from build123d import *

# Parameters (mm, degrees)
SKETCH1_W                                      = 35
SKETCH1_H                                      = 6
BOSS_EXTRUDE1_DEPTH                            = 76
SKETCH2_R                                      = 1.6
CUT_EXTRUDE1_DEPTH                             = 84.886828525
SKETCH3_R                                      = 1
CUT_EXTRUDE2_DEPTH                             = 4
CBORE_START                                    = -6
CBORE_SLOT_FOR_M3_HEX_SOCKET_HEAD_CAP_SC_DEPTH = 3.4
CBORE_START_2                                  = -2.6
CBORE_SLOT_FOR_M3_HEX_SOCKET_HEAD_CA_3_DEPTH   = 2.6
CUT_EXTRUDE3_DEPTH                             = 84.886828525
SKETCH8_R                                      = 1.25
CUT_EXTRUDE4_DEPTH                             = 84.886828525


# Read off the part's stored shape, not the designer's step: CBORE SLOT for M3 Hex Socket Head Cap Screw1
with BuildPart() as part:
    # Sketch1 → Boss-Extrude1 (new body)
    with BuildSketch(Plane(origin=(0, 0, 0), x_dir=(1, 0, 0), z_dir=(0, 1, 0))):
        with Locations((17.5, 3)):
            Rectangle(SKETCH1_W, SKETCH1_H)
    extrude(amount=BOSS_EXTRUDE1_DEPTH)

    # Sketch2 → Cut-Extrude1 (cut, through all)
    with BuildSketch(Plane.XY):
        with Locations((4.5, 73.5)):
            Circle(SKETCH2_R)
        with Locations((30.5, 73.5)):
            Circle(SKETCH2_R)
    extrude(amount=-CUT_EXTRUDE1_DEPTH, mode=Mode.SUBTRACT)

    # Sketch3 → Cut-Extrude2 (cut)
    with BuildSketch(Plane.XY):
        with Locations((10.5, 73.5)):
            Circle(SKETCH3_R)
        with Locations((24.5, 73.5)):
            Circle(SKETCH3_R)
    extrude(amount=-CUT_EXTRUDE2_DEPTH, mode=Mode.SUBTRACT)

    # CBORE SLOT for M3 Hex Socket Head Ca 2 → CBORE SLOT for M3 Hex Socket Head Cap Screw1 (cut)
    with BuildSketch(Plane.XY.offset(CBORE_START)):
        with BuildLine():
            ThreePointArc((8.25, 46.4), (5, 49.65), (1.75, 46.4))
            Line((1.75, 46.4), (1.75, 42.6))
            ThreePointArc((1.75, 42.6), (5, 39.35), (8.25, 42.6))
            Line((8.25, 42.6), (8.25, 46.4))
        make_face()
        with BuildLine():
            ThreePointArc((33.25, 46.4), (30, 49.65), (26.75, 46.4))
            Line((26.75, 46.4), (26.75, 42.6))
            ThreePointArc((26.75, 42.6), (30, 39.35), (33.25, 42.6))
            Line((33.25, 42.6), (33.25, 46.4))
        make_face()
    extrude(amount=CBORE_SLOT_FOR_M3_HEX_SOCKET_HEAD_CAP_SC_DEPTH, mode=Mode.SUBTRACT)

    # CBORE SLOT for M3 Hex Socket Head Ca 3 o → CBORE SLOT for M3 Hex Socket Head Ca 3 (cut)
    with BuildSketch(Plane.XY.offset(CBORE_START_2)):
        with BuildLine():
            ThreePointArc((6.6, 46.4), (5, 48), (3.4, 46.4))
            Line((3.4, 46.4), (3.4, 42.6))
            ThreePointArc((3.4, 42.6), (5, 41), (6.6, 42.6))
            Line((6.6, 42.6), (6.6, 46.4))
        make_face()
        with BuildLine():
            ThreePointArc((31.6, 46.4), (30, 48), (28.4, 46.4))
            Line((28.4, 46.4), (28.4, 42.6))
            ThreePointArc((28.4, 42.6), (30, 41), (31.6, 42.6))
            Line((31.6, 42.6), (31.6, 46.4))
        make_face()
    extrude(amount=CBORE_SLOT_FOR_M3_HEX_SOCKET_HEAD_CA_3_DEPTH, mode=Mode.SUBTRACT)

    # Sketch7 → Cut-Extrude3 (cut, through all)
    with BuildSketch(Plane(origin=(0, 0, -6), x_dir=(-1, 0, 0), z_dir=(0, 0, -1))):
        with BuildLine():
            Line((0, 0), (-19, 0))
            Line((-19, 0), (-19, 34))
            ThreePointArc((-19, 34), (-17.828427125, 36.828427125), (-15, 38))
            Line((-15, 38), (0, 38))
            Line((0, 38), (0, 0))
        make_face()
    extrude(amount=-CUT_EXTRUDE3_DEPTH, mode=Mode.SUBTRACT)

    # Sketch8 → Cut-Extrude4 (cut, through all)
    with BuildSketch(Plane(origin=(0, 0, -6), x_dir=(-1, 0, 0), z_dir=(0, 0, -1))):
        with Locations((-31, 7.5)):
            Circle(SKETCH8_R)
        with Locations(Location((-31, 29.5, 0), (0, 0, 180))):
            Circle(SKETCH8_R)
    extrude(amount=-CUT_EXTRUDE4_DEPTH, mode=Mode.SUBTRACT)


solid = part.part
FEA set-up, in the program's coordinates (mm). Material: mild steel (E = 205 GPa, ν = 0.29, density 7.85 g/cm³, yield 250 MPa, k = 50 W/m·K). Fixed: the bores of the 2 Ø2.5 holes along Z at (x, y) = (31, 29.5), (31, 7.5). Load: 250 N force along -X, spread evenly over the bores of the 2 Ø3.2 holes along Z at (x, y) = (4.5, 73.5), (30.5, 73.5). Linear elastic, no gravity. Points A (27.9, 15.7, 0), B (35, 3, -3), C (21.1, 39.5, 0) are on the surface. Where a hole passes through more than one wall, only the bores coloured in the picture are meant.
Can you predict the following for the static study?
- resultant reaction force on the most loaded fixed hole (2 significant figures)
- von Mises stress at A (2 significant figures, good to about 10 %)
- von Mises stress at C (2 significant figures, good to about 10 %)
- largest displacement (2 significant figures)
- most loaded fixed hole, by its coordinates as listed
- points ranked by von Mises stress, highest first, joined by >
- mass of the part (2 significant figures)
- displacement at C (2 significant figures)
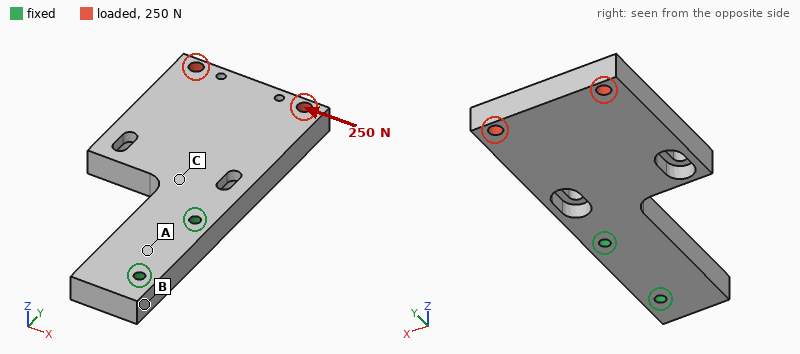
800 N
12 MPa
20 MPa
31 µm
(31, 29.5)
C > A > B
86 g
4.8 µm
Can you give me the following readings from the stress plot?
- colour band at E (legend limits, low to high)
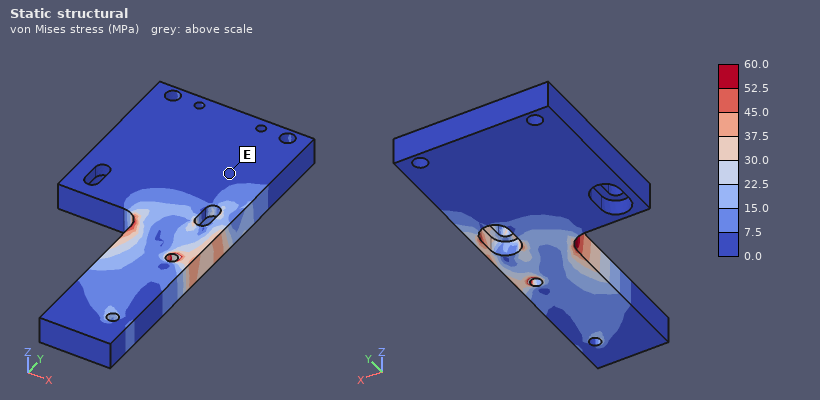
0.0 to 7.5 MPa
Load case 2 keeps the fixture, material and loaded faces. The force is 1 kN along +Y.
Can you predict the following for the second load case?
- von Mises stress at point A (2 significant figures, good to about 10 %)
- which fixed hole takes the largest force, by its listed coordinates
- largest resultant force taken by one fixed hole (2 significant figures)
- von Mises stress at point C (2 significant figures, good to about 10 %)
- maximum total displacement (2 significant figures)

16 MPa
(31, 7.5)
820 N
26 MPa
31 µm
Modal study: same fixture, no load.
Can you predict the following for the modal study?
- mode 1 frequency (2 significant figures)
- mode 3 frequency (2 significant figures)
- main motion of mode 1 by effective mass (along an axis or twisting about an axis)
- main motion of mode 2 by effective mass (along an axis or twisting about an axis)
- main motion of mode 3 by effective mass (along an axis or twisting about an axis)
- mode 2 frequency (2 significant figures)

1300 Hz
3600 Hz
along Z
along X
twisting about Y
2900 Hz
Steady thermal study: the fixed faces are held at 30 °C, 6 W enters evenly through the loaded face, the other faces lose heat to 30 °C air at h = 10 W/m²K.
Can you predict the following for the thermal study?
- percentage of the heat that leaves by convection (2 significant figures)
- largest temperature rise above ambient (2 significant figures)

18 %
42 K
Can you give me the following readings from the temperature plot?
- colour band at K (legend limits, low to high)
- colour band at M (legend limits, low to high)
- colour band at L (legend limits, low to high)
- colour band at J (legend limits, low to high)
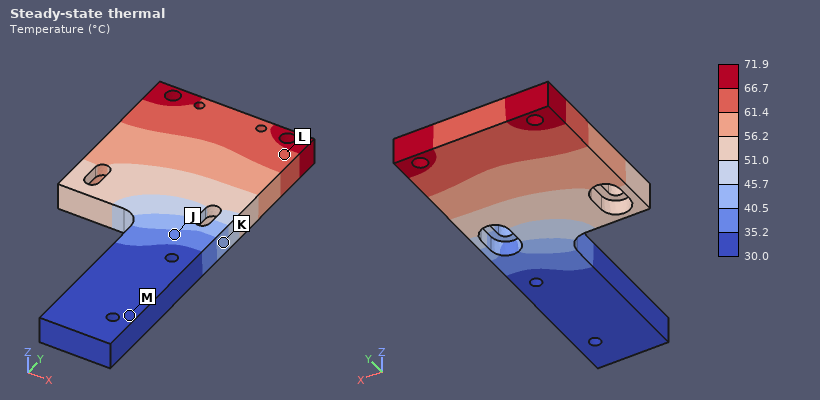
40.5 to 45.7 °C
30.0 to 35.2 °C
61.4 to 66.7 °C
35.2 to 40.5 °C
